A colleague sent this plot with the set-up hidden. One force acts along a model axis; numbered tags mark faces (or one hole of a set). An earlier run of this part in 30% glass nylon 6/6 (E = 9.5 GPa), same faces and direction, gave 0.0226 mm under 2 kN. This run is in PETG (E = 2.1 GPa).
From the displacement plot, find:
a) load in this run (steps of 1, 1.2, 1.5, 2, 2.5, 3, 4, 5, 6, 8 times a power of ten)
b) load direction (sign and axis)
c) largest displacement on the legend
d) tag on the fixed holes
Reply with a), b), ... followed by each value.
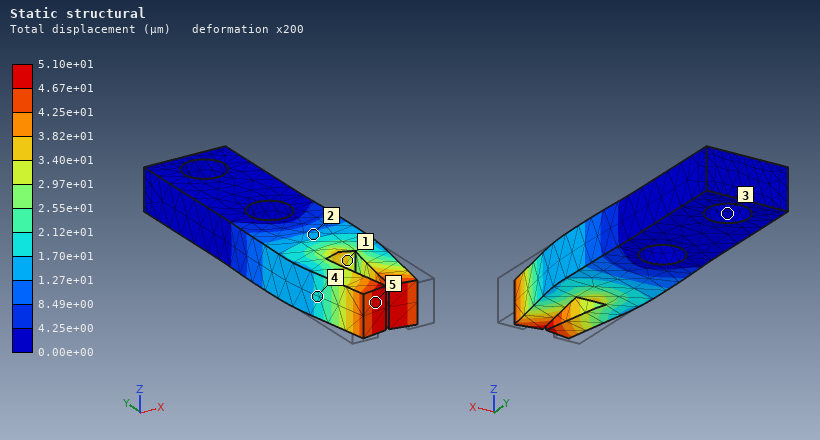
a) 1 kN
b) +Y
c) 5.10e+01 µm
d) 3
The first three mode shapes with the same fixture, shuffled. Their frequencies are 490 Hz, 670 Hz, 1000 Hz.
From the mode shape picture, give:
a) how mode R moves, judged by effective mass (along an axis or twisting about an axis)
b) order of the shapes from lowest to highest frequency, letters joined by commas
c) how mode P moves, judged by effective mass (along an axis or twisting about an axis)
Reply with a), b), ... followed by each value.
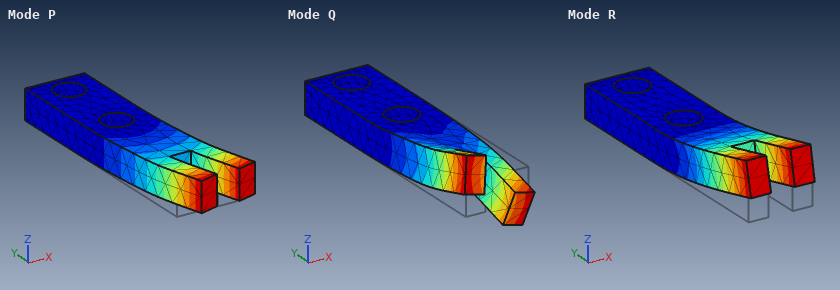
a) along Z
b) R, P, Q
c) along X
